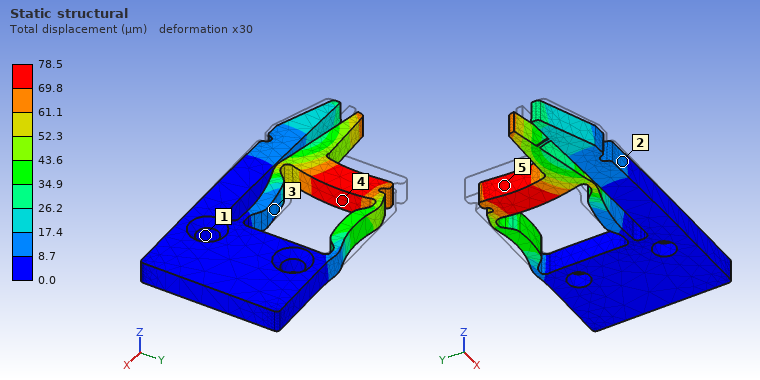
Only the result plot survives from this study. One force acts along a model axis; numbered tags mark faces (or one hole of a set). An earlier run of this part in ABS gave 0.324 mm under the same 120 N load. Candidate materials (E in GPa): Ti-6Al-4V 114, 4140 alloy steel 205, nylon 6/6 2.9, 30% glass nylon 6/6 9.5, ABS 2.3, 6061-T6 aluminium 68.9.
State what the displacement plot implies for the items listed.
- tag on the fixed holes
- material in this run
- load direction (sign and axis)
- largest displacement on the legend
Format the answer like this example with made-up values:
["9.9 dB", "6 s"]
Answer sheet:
["1", "30% glass nylon 6/6", "+X", "78.5 µm"]
